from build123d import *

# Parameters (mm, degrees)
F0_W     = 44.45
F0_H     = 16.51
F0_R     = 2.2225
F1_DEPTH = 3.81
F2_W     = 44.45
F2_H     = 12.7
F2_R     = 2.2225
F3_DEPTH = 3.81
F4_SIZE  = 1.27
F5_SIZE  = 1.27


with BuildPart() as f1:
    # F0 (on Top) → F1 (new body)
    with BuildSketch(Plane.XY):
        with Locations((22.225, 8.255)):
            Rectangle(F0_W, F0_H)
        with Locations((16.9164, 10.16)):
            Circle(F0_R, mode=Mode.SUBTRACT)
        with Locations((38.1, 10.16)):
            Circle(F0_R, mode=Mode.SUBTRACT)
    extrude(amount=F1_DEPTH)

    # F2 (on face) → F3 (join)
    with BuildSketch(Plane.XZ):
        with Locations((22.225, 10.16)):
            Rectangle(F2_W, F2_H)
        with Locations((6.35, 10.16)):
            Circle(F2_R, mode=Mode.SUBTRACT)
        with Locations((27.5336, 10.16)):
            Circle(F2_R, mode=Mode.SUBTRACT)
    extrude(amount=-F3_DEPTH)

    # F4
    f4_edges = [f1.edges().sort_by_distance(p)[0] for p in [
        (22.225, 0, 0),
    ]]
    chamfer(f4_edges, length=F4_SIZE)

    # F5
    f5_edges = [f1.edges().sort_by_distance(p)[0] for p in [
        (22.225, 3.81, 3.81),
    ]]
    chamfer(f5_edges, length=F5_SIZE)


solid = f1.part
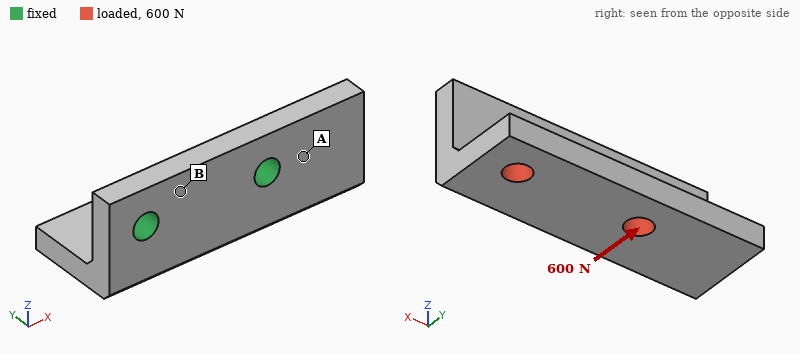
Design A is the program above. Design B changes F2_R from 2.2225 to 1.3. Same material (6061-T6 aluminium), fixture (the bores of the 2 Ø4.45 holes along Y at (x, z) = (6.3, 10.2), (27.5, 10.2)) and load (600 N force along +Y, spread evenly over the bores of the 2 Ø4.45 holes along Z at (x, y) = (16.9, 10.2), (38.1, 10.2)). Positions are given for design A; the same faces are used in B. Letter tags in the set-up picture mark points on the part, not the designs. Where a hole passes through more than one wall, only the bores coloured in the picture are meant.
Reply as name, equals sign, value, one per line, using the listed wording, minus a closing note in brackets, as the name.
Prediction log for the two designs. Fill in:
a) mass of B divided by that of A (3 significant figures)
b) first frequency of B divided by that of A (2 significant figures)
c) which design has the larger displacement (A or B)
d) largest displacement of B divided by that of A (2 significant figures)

mass of B divided by that of A = 1.02
first frequency of B divided by that of A = 0.86
which design has the larger displacement = B
largest displacement of B divided by that of A = 1.4
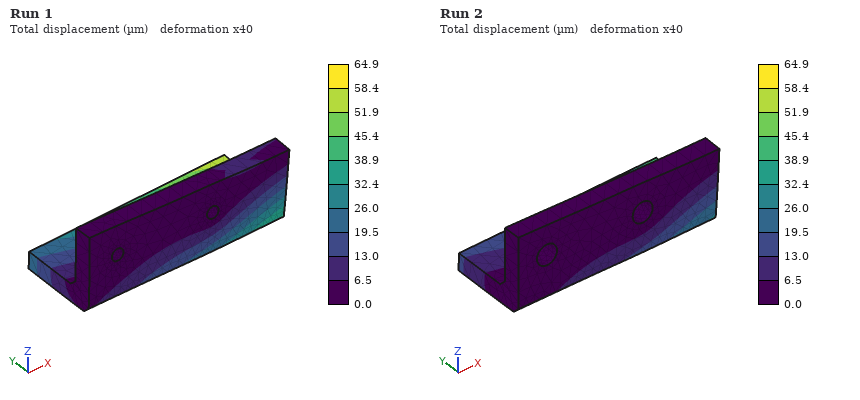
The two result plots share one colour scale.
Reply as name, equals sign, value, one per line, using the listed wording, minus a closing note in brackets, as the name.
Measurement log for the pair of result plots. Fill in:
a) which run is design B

which run is design B = Run 1
